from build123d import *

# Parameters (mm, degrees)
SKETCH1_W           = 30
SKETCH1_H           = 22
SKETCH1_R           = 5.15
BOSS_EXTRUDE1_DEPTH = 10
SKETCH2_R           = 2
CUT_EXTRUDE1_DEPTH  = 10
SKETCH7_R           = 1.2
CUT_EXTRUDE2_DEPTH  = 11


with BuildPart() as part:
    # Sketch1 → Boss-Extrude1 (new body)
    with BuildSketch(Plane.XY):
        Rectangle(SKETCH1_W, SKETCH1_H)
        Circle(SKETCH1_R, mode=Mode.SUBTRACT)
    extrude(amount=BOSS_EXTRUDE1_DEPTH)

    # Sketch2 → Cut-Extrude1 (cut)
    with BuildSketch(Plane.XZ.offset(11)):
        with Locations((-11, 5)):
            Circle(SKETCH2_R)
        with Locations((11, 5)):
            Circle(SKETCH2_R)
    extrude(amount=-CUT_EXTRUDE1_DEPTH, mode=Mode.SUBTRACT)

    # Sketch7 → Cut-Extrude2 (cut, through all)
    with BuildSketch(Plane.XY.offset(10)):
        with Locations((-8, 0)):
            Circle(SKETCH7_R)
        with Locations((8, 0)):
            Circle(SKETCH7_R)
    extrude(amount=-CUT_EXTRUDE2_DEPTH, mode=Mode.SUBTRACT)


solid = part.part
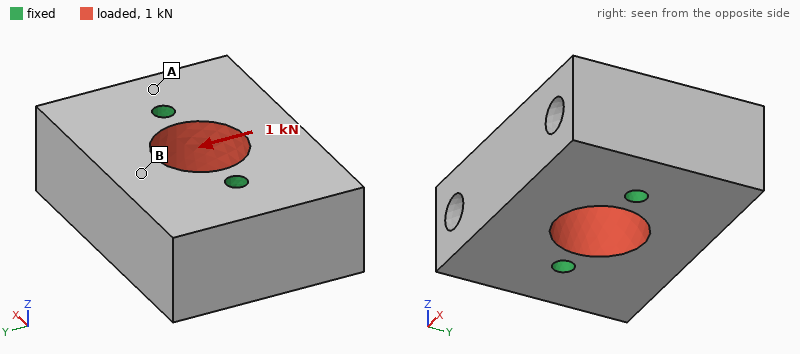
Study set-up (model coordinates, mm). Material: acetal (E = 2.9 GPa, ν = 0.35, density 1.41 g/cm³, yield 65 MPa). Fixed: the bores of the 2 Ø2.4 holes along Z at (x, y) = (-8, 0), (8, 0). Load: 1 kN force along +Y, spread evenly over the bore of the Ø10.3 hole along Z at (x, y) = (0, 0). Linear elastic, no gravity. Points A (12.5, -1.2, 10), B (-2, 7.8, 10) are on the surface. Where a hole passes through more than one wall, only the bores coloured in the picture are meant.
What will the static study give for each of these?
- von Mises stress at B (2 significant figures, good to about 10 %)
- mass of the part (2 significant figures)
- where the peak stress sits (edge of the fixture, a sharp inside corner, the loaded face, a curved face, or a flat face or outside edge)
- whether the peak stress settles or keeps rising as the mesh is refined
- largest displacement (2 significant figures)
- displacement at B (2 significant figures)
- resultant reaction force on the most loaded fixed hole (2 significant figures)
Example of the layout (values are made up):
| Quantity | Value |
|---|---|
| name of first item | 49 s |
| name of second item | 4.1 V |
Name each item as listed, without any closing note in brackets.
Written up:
| Quantity | Value |
|---|---|
| von Mises stress at B | 3.6 MPa |
| mass of the part | 7.6 g |
| where the peak stress sits | edge of the fixture |
| whether the peak stress settles or keeps rising as the mesh is refined | keeps rising |
| largest displacement | 22 µm |
| displacement at B | 18 µm |
| resultant reaction force on the most loaded fixed hole | 500 N |
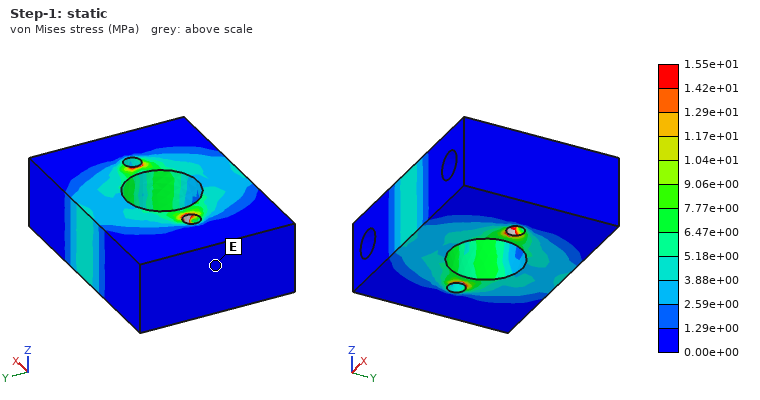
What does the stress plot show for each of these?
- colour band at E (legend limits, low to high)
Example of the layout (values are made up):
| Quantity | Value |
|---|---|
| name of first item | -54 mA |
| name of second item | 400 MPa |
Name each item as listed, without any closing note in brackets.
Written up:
| Quantity | Value |
|---|---|
| colour band at E | 0.00e+00 to 1.29e+00 MPa |
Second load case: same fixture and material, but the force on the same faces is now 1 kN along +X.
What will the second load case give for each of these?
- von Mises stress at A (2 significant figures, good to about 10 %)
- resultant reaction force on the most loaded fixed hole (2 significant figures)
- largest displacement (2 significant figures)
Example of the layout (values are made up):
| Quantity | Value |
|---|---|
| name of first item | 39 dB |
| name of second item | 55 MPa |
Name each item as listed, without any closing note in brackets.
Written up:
| Quantity | Value |
|---|---|
| von Mises stress at A | 2.4 MPa |
| resultant reaction force on the most loaded fixed hole | 500 N |
| largest displacement | 21 µm |
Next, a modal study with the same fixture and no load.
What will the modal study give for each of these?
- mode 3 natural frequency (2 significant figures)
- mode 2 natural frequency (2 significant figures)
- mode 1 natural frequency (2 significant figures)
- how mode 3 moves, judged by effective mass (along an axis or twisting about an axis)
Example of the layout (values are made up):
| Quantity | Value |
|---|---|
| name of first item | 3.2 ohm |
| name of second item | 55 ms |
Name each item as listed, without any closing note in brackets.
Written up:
| Quantity | Value |
|---|---|
| mode 3 natural frequency | 11 kHz |
| mode 2 natural frequency | 9400 Hz |
| mode 1 natural frequency | 9000 Hz |
| how mode 3 moves, judged by effective mass | along Z |
